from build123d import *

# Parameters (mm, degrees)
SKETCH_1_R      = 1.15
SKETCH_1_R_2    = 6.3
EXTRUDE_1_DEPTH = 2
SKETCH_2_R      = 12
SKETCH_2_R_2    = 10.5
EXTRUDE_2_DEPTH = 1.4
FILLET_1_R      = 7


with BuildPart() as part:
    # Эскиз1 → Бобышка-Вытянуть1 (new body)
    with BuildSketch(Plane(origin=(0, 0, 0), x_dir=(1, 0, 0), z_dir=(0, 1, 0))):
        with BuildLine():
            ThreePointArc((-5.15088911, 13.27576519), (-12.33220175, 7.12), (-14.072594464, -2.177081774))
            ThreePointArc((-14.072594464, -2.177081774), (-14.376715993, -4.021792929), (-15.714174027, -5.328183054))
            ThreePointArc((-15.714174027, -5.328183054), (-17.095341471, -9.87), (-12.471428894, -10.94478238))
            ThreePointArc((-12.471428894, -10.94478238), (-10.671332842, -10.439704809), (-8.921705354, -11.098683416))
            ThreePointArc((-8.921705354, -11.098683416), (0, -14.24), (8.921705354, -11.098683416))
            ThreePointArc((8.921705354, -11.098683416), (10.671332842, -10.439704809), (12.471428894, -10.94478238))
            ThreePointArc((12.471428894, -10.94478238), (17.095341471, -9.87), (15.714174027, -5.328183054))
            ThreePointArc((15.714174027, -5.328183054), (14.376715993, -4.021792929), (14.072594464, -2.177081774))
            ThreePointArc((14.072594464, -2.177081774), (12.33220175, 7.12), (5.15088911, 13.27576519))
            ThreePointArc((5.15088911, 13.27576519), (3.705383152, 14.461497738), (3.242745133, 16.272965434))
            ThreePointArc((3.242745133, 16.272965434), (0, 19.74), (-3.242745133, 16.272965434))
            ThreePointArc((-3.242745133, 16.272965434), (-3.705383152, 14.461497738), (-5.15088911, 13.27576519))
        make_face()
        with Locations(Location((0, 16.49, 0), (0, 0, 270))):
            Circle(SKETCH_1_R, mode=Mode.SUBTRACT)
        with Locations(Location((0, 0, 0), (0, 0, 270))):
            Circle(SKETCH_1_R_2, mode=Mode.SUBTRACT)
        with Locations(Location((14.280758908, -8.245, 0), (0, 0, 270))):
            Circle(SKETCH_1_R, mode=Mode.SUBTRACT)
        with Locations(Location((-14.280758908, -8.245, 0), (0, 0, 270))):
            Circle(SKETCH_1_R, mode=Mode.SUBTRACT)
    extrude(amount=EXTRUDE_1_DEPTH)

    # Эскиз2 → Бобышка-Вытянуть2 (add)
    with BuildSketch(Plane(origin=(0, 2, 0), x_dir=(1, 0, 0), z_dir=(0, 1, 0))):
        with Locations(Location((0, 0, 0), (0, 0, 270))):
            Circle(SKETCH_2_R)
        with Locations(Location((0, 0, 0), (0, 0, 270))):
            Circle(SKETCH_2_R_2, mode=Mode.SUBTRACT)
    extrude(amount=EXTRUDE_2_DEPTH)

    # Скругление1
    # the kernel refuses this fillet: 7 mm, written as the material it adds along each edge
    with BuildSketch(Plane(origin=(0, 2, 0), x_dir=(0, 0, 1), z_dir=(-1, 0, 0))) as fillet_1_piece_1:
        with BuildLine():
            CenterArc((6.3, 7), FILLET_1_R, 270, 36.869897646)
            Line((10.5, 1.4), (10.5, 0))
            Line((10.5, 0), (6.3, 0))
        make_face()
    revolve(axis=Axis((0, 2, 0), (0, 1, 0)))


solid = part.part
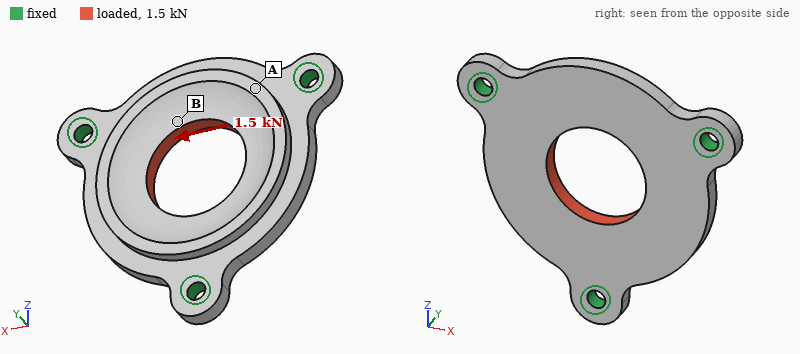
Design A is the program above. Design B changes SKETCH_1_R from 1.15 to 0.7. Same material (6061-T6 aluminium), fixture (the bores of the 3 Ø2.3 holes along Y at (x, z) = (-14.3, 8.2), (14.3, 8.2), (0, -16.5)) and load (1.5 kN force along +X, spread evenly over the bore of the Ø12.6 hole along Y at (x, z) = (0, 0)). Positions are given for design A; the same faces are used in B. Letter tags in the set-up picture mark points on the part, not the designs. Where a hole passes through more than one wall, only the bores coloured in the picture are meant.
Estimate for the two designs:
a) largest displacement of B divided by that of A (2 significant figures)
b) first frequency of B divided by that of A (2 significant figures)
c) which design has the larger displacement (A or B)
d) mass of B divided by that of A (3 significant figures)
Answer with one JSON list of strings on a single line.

["1.1", "0.90", "B", "1.01"]
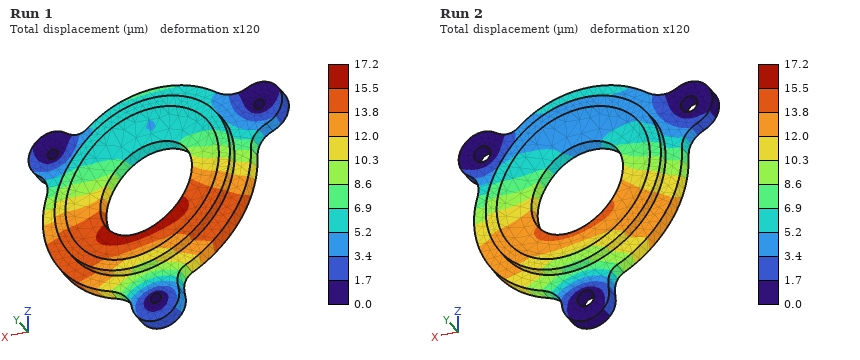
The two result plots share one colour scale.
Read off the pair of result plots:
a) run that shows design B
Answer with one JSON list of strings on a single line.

["Run 1"]
